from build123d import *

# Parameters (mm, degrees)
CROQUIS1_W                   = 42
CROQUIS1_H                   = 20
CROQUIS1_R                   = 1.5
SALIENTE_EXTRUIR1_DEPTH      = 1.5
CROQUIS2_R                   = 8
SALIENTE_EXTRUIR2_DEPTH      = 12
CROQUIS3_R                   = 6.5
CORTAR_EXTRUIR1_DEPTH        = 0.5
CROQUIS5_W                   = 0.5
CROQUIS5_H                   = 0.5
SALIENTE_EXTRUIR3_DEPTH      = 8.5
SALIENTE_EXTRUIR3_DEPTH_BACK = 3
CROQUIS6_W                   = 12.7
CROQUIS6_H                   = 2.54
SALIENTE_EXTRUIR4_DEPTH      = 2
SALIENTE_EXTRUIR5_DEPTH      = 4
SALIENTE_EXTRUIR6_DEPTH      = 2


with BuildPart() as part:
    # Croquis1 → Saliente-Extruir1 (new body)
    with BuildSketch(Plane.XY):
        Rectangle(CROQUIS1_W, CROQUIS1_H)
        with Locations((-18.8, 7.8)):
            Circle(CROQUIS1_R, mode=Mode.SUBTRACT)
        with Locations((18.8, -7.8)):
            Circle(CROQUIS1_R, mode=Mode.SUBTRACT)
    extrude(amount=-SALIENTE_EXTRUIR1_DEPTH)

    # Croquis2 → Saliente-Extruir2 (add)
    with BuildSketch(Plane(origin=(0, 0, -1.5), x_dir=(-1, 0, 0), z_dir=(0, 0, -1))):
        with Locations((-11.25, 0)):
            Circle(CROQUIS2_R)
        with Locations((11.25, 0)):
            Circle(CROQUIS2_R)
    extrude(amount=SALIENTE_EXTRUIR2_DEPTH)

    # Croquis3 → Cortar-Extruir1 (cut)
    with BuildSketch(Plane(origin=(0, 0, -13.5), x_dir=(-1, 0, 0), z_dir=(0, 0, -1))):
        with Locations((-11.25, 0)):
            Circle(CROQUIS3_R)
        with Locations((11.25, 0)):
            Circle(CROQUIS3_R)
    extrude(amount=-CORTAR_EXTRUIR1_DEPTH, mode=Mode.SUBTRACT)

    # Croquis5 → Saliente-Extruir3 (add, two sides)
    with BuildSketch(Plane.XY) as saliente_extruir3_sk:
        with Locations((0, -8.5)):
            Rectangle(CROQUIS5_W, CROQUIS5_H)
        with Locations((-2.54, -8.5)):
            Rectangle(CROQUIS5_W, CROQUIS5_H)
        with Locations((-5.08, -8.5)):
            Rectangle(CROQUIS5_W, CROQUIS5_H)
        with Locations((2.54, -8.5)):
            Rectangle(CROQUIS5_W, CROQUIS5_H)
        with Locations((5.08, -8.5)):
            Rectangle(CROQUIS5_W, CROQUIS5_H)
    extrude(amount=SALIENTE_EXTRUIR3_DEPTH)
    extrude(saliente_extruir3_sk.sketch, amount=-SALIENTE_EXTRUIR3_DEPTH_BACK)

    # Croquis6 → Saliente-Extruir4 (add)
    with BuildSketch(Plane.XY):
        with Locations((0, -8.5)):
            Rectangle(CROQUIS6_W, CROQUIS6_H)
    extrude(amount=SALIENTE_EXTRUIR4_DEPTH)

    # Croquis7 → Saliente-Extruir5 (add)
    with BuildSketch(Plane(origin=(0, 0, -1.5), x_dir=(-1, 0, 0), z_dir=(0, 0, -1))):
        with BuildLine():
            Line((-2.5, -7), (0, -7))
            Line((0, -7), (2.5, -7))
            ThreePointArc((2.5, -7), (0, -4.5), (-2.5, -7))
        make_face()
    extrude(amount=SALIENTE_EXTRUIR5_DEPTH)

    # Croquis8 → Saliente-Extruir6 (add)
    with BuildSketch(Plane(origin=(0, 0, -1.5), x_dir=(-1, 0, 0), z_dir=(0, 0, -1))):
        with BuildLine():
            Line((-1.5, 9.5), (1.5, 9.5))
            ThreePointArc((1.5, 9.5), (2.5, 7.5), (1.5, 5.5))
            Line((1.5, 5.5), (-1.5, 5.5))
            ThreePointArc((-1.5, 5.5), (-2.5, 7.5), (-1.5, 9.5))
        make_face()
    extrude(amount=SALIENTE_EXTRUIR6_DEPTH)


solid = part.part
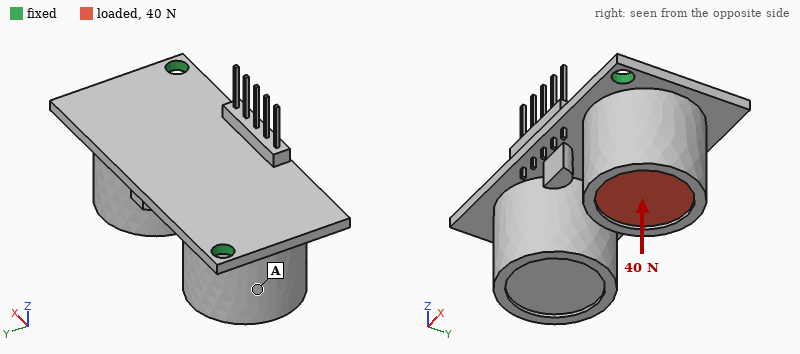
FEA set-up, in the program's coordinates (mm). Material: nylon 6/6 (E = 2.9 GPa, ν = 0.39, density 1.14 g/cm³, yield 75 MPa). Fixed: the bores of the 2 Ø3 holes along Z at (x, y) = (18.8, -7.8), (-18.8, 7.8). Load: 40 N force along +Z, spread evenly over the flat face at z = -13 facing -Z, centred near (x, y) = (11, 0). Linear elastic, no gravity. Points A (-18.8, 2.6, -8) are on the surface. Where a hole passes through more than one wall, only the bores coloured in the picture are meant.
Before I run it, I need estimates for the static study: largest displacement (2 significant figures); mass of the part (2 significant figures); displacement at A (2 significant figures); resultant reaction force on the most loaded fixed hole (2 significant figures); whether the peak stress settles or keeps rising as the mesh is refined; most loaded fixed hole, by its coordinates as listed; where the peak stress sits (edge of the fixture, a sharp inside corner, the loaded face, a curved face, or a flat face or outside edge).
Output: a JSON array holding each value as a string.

["0.52 mm", "6.9 g", "0.13 mm", "31 N", "keeps rising", "(18.8, -7.8)", "edge of the fixture"]
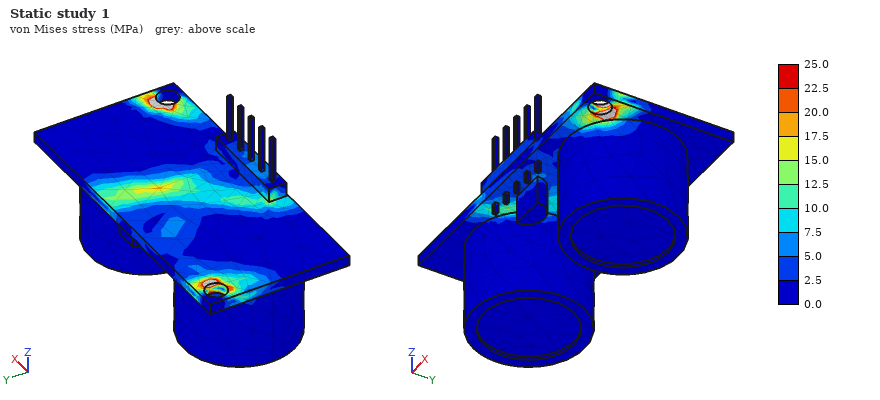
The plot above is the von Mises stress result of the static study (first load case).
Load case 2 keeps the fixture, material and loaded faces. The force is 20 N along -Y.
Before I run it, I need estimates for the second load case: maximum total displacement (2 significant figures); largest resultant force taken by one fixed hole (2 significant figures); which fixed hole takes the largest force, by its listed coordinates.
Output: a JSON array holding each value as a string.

["0.52 mm", "17 N", "(18.8, -7.8)"]
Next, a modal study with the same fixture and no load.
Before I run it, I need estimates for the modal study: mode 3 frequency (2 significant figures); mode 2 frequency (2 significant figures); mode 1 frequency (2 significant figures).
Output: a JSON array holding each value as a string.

["1300 Hz", "740 Hz", "710 Hz"]
